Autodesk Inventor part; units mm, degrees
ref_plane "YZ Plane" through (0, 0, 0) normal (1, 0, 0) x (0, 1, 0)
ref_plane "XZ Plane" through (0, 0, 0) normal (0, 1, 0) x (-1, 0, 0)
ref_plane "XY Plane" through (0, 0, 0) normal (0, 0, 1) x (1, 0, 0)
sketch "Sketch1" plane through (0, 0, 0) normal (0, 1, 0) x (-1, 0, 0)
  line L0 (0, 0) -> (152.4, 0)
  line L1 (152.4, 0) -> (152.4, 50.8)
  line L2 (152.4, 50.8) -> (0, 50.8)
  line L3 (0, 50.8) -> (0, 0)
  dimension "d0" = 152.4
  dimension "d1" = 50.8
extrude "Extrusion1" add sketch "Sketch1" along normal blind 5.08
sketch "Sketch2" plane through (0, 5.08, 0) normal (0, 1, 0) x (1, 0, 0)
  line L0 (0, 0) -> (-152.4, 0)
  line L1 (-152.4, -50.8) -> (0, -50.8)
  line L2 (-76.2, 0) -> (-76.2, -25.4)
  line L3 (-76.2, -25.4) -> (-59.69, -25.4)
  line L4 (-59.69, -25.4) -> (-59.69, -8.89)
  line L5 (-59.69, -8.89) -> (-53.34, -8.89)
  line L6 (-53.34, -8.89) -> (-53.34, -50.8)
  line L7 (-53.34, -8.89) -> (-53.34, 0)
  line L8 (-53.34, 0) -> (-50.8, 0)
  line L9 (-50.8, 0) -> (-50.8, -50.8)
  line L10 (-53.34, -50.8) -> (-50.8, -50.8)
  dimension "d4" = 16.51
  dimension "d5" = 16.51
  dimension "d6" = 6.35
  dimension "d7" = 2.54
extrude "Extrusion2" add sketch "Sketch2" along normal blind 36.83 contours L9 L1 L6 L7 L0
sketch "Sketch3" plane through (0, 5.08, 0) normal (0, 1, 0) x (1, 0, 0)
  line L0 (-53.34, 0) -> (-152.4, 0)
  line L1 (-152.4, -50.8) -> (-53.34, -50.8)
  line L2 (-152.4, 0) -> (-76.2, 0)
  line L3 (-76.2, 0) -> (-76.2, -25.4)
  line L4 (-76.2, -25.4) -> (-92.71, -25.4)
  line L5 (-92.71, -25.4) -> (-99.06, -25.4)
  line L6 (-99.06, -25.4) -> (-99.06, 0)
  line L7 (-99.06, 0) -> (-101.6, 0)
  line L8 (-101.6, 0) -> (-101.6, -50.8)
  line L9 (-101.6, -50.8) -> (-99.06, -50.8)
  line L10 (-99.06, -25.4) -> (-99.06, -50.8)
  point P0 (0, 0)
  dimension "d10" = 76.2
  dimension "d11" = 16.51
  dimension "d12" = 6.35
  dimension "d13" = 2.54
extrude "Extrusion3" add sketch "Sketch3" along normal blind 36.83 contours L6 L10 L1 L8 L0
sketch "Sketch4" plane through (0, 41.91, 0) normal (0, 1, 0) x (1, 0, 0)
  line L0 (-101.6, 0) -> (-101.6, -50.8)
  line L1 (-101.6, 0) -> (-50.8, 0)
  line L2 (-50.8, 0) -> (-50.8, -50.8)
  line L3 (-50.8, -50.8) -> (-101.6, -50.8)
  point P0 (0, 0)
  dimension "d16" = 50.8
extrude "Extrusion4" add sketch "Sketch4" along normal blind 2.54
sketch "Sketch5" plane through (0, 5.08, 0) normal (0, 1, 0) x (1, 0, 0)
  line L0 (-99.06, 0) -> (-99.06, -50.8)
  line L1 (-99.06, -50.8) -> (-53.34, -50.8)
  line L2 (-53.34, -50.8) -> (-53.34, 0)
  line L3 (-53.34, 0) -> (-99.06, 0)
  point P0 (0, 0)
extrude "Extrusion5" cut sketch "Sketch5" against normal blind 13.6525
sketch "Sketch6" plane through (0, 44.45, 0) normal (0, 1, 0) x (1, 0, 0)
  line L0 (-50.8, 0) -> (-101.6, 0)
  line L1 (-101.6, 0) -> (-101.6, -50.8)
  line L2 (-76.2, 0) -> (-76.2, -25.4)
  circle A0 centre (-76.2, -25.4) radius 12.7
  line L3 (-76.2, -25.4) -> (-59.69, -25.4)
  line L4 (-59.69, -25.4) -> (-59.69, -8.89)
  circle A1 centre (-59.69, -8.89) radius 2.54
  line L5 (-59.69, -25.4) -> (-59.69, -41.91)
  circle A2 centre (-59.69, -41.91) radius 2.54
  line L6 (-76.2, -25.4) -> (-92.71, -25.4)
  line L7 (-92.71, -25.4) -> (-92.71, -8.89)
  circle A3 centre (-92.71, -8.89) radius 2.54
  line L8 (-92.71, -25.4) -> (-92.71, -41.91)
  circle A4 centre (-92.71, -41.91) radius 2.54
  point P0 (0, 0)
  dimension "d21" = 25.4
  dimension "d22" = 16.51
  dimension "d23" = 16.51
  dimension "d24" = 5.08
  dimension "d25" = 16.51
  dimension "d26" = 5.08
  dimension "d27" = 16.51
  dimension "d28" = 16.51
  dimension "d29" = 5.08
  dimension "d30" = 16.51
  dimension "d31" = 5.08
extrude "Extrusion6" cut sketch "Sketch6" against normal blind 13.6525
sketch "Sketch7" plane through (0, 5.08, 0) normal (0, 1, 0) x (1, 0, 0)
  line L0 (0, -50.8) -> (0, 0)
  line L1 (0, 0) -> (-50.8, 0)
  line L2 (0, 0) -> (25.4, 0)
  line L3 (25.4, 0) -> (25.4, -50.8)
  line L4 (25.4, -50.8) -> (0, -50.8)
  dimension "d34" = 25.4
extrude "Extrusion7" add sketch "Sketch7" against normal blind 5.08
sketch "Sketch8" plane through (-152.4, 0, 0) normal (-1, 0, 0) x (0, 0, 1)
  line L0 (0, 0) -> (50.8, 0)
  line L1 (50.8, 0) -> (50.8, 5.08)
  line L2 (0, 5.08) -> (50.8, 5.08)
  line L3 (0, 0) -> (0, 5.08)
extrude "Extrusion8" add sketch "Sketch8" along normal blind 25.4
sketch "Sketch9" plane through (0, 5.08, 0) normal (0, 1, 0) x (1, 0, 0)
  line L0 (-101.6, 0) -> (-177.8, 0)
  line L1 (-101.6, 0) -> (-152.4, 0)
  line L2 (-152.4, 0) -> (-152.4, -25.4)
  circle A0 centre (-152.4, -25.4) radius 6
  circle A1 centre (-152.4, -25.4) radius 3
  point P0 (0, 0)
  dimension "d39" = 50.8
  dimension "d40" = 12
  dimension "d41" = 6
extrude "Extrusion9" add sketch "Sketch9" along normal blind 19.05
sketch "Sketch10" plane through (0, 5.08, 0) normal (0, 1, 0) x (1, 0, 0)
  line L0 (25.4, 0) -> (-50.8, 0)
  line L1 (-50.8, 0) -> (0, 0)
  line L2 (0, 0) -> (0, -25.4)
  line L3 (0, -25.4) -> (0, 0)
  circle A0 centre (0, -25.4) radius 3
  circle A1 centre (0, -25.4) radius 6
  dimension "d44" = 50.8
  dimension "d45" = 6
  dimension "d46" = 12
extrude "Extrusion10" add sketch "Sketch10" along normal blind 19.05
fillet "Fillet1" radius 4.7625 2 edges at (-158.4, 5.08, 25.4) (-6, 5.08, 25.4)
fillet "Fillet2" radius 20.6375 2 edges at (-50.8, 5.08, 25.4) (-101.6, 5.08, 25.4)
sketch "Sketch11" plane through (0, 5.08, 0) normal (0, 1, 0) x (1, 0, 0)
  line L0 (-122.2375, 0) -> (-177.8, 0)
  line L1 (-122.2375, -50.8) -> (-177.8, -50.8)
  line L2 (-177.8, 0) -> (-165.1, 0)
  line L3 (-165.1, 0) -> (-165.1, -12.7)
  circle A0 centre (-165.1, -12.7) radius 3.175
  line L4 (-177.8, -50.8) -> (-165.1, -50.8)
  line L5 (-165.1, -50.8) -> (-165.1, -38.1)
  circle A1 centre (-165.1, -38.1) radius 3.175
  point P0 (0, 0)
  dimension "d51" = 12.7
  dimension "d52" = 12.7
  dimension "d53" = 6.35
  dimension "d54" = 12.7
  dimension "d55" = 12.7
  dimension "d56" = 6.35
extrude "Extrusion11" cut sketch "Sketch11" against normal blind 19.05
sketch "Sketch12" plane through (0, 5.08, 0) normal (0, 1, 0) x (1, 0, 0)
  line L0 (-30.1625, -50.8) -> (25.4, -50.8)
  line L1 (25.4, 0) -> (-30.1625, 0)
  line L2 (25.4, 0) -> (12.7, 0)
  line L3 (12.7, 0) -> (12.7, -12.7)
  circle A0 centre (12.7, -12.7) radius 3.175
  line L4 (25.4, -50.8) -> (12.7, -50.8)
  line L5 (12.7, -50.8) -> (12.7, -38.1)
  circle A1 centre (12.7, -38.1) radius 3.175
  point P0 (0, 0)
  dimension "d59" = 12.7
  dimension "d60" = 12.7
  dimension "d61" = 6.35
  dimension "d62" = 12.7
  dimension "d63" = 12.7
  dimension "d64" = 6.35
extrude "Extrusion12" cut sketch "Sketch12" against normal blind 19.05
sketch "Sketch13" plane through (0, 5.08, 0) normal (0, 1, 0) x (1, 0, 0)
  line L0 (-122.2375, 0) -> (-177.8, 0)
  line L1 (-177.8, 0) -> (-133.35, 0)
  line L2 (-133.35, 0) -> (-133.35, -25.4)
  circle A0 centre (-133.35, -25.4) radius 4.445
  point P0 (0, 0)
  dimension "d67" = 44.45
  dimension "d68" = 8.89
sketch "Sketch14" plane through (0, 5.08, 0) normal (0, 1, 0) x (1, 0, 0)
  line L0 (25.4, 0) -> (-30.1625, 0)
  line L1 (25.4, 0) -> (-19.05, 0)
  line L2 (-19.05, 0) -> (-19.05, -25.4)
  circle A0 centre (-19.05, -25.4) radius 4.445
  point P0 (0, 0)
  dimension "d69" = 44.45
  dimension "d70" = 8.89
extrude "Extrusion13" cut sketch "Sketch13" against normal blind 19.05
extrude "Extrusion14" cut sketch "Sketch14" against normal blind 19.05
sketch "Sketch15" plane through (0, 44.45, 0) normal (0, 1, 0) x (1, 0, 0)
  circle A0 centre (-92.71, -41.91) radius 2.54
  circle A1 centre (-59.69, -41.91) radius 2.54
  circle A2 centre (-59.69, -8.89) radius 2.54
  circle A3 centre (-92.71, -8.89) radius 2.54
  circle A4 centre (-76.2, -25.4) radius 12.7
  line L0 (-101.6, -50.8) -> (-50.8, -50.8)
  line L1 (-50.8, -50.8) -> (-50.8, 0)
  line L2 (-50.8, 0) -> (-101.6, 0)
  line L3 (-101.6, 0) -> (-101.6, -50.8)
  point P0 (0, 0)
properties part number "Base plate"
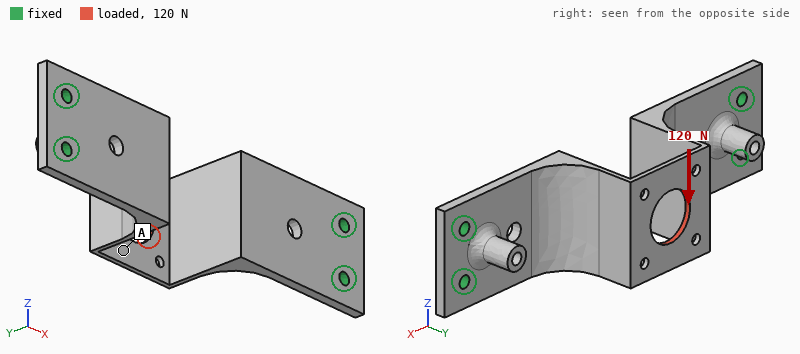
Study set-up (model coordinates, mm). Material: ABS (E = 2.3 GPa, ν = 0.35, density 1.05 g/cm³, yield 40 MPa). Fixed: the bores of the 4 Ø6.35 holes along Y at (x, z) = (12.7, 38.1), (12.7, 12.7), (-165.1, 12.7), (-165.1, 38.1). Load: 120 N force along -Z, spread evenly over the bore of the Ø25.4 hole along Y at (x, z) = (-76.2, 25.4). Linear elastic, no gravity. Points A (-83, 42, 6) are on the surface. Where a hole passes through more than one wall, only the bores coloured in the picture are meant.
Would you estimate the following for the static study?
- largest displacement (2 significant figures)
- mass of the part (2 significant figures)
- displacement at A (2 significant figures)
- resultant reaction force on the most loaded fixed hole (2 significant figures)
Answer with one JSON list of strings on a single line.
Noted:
["2.1 mm", "70 g", "1.9 mm", "170 N"]
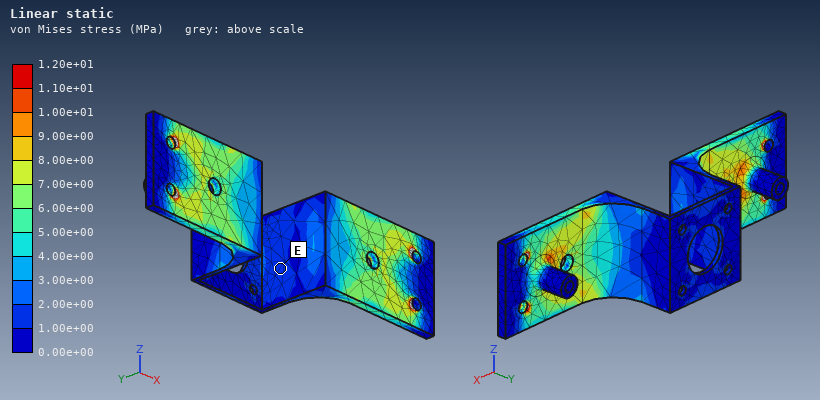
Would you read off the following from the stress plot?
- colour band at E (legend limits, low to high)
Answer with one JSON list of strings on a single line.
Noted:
["1.00e+00 to 2.00e+00 MPa"]
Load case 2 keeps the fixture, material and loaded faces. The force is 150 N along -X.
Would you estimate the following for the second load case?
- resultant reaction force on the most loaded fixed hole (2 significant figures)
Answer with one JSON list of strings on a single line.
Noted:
["42 N"]
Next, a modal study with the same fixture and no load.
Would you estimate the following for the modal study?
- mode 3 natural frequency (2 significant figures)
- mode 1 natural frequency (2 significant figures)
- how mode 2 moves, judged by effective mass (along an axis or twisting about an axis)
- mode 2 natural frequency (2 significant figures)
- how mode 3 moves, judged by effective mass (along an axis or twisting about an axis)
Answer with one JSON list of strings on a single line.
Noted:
["350 Hz", "250 Hz", "along Y", "260 Hz", "along Z"]
